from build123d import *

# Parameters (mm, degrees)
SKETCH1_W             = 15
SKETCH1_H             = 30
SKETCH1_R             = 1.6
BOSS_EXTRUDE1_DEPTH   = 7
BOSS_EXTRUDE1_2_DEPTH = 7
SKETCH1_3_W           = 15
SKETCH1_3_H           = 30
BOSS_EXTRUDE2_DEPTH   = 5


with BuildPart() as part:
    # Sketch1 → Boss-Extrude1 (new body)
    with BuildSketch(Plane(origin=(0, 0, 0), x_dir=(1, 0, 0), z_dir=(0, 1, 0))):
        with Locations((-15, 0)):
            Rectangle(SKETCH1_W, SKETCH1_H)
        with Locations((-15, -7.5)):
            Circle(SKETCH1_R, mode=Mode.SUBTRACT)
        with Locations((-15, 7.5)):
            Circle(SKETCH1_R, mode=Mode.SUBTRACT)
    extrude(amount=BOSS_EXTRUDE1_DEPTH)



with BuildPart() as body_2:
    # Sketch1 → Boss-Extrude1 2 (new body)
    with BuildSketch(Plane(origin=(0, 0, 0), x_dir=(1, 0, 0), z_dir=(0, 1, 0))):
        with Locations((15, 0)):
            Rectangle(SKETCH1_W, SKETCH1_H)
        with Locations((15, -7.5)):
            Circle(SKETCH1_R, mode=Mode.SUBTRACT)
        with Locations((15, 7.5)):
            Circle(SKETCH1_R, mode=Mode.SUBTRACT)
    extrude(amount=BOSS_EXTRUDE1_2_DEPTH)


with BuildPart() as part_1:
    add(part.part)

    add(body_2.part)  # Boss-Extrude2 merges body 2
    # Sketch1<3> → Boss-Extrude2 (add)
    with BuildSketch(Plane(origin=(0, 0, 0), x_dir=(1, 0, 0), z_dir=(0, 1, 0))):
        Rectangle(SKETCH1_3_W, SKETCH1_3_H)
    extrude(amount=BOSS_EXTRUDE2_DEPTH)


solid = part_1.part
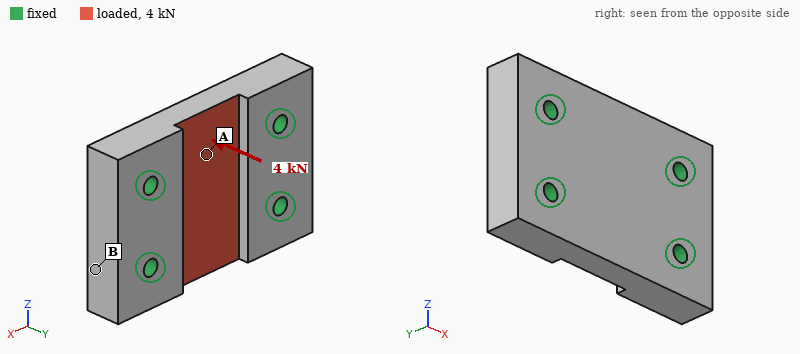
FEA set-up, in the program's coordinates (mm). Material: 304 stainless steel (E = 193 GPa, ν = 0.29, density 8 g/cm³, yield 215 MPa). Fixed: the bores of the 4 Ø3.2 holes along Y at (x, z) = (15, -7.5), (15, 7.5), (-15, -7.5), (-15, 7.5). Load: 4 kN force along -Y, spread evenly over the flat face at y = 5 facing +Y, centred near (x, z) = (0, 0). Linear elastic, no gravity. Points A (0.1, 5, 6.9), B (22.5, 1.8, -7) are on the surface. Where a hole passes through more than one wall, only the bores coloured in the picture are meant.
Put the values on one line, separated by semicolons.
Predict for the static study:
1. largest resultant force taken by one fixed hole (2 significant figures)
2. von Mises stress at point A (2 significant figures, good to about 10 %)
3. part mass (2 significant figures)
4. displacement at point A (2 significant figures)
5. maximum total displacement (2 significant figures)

1.1 kN; 37 MPa; 67 g; 6.3 µm; 7.2 µm
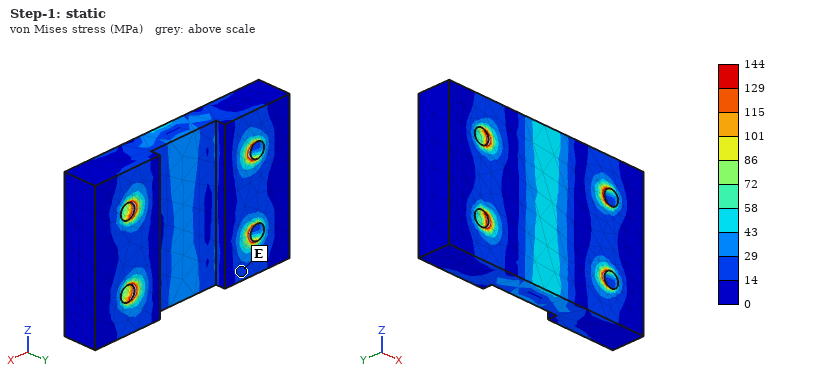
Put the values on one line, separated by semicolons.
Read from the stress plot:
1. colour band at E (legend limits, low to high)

14 to 29 MPa
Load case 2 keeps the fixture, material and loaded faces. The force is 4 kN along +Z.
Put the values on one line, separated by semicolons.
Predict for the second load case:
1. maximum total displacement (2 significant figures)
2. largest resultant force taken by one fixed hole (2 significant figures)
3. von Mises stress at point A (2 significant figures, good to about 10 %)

4.0 µm; 1.1 kN; 18 MPa
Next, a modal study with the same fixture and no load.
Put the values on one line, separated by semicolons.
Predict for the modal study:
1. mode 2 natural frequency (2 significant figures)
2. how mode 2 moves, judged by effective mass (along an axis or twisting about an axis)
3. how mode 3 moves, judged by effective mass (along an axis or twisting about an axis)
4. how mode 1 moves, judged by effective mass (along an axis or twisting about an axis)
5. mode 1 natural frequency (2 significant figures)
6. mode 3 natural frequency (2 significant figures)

32 kHz; twisting about X; along Z; along Y; 29 kHz; 46 kHz
